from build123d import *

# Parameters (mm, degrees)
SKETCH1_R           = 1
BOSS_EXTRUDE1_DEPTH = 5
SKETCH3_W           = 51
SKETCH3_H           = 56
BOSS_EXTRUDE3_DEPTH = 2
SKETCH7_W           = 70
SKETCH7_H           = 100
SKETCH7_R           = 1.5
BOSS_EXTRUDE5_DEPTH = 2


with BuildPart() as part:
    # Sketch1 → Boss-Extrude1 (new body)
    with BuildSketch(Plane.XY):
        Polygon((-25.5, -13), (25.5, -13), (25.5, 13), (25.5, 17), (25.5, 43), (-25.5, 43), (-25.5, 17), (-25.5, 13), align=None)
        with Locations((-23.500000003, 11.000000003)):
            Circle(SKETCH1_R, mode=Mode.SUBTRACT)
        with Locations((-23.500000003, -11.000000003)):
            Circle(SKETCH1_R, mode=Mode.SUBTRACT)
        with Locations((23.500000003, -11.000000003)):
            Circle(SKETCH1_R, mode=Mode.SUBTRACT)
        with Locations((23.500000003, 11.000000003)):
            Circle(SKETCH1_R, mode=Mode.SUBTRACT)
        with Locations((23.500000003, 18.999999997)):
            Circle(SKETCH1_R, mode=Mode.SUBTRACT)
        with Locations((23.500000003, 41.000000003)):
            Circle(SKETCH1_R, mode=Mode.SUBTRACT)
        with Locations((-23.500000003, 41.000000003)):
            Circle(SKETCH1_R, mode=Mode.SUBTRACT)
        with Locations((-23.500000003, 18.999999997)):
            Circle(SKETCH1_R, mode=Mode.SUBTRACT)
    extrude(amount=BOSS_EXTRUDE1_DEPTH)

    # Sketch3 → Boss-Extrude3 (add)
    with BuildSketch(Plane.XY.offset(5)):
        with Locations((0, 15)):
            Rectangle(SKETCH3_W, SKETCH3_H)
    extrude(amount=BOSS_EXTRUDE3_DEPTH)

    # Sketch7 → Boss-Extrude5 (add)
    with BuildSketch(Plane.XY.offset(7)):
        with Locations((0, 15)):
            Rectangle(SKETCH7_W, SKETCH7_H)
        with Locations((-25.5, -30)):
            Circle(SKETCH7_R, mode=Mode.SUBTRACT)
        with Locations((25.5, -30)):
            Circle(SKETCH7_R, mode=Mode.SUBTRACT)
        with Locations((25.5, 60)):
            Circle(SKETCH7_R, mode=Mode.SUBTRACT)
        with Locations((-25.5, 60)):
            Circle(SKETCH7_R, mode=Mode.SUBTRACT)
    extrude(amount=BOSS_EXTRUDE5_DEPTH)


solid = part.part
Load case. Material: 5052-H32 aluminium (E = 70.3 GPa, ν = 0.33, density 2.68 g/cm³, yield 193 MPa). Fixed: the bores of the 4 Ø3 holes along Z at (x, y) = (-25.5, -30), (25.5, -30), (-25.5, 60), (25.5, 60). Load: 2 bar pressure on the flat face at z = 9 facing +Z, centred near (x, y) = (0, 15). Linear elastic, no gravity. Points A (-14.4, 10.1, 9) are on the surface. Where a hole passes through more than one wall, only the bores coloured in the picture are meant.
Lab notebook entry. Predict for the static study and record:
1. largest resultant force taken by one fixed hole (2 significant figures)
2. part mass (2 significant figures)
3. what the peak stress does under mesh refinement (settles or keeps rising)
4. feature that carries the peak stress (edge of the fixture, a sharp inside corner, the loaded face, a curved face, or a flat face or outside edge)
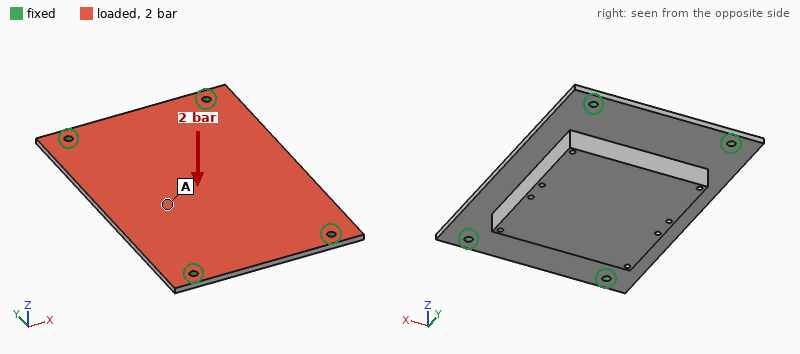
430 N
91 g
keeps rising
edge of the fixture
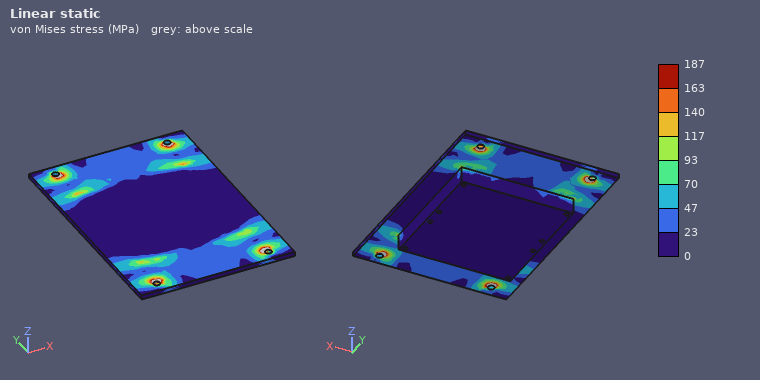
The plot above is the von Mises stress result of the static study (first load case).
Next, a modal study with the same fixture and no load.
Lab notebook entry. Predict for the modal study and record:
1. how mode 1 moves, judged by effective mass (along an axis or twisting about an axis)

along Z
